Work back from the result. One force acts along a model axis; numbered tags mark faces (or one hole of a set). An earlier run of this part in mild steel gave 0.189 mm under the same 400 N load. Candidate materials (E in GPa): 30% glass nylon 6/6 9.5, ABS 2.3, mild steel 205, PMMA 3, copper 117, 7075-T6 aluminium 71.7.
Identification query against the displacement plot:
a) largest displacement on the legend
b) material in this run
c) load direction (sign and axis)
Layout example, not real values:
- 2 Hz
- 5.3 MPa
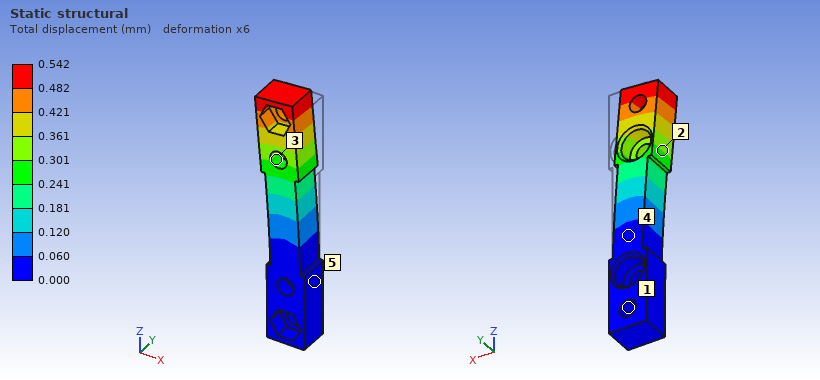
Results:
- 0.542 mm
- 7075-T6 aluminium
- -X
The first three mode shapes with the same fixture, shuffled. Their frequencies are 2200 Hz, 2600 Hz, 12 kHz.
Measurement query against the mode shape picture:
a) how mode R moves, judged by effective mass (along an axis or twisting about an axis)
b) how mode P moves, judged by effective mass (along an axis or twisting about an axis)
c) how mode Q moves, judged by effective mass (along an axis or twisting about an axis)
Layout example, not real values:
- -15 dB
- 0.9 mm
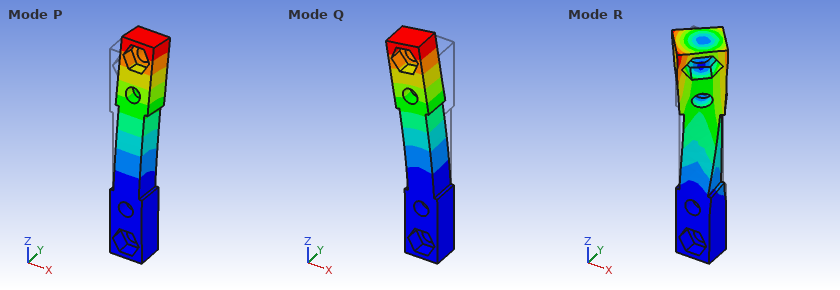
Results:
- twisting about Z
- along Y
- along X
